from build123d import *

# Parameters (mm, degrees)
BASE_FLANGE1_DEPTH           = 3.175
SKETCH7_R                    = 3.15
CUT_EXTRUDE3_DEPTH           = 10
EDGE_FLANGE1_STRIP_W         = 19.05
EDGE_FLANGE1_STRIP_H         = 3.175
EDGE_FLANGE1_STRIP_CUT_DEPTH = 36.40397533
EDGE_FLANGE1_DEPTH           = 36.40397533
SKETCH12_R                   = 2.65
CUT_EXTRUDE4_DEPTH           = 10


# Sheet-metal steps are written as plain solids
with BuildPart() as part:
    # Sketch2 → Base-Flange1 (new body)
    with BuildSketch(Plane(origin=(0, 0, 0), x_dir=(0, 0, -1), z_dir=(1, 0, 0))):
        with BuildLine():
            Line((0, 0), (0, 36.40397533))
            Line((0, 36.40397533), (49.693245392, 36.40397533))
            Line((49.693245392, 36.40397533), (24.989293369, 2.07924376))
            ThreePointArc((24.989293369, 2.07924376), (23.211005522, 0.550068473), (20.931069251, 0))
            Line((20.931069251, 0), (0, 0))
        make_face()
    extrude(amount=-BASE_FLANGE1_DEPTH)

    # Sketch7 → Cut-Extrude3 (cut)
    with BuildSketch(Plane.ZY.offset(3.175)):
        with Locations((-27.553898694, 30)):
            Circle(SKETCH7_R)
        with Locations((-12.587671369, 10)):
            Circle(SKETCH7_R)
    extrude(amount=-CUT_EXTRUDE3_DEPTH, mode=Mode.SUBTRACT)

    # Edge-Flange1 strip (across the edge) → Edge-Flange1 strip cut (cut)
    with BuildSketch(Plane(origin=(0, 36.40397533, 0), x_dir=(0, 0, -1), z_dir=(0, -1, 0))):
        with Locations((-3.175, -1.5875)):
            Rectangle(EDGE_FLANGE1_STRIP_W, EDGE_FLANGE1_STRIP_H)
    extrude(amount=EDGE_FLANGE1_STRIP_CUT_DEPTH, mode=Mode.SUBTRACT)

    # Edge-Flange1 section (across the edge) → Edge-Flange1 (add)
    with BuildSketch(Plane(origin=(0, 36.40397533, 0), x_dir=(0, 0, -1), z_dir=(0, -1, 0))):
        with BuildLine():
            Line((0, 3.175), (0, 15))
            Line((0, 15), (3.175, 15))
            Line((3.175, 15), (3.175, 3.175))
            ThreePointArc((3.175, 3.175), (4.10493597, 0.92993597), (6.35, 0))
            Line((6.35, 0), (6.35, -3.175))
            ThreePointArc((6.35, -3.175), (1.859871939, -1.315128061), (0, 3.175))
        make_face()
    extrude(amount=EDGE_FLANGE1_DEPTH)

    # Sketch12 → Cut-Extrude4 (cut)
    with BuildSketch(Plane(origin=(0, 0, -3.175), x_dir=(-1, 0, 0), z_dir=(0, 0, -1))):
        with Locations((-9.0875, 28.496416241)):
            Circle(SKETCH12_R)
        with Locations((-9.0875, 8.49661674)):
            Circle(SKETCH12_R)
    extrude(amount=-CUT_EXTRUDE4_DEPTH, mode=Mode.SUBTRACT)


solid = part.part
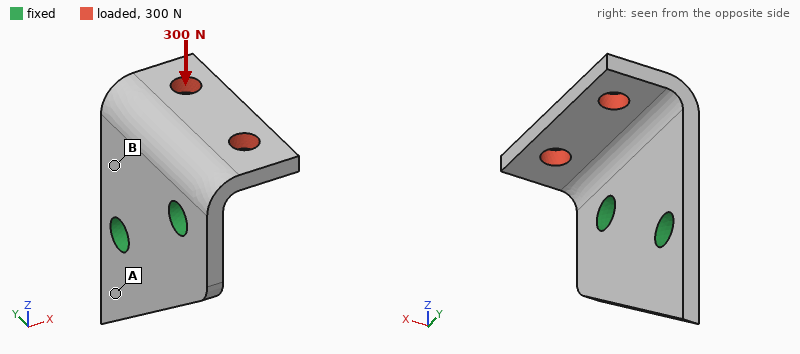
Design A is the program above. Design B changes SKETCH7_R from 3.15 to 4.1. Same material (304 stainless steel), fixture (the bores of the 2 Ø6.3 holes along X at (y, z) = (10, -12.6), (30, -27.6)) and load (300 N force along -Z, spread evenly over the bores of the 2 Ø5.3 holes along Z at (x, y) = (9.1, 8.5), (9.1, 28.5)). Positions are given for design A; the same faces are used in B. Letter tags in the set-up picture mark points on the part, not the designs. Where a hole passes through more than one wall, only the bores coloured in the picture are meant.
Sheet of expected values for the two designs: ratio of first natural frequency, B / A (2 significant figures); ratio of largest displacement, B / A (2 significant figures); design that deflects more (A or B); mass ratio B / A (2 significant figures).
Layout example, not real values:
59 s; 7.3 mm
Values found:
1.1; 0.90; A; 0.97
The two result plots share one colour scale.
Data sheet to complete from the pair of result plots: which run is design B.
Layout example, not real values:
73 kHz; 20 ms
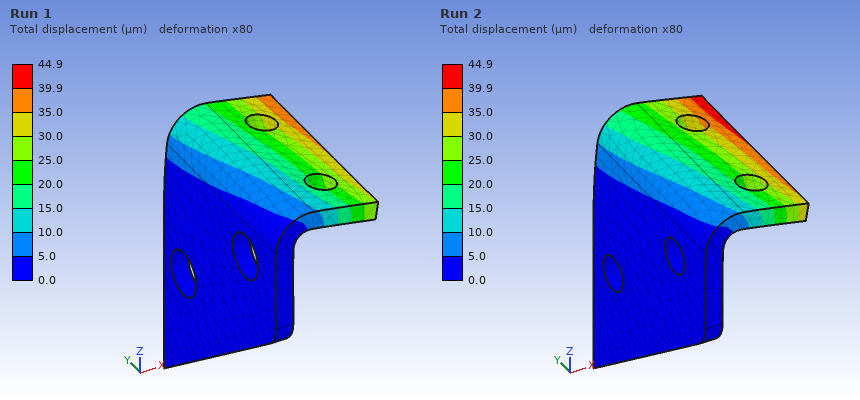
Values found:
Run 1
